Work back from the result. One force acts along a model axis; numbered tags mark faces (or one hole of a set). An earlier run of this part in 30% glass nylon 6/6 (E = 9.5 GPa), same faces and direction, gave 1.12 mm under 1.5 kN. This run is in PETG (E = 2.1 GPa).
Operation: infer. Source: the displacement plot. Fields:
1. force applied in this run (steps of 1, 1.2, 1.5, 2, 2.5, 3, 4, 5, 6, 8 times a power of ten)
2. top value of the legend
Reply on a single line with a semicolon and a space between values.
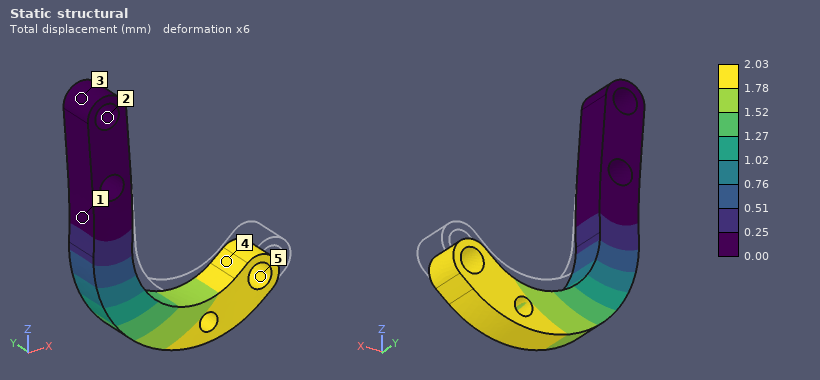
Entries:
600 N; 2.03 mm
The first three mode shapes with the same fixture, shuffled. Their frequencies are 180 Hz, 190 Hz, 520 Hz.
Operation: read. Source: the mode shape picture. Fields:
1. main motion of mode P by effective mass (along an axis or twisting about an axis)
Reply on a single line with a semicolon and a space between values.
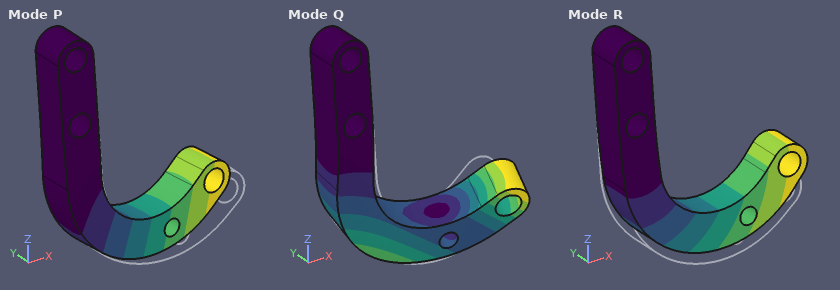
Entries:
along Y
